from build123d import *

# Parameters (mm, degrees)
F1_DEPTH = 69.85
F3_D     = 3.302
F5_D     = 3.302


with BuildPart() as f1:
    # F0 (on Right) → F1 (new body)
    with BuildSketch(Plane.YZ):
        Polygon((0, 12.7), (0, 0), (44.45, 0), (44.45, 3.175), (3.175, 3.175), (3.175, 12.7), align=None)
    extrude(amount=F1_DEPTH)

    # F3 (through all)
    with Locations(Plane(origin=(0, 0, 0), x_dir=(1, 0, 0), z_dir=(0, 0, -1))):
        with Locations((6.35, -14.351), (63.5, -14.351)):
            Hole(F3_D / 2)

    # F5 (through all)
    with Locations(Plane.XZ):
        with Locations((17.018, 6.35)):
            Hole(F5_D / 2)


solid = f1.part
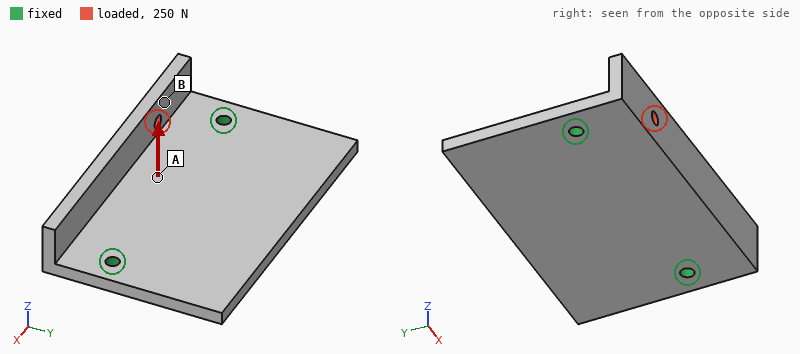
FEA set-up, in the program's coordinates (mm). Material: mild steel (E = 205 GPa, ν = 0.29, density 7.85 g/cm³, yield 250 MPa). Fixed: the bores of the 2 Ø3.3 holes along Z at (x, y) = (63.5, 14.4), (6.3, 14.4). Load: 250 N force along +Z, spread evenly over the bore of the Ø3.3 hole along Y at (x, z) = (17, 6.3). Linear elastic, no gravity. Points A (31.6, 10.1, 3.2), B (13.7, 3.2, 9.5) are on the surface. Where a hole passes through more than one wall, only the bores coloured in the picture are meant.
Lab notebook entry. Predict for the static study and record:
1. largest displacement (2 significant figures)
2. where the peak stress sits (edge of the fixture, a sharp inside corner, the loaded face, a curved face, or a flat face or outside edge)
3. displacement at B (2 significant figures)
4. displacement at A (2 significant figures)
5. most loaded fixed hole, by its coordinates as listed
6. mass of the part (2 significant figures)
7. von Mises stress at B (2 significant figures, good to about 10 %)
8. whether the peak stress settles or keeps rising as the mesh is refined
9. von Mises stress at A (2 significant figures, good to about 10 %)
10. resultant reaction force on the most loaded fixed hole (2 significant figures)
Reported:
21 µm
edge of the fixture
15 µm
5.4 µm
(6.3, 14.4)
93 g
17 MPa
keeps rising
7.7 MPa
210 N
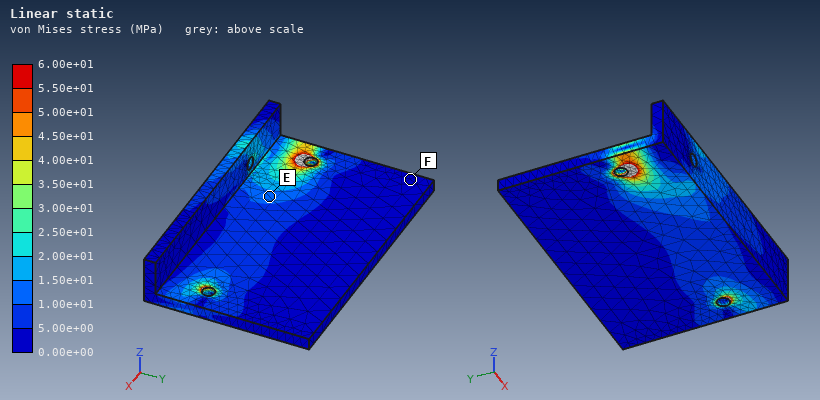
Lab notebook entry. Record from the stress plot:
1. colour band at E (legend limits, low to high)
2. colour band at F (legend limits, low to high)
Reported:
1.00e+01 to 1.50e+01 MPa
0.00e+00 to 5.00e+00 MPa
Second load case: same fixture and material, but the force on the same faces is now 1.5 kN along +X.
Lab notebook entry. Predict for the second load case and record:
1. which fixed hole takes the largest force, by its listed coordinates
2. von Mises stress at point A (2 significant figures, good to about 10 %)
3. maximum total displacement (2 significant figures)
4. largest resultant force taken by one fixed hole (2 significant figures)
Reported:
(6.3, 14.4)
16 MPa
13 µm
930 N
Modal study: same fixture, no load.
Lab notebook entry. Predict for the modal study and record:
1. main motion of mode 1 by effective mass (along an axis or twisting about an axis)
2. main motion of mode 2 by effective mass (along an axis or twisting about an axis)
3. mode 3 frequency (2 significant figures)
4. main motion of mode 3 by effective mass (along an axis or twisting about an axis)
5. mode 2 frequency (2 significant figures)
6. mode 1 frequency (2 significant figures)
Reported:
along Z
twisting about Y
4600 Hz
along Z
4000 Hz
2100 Hz
